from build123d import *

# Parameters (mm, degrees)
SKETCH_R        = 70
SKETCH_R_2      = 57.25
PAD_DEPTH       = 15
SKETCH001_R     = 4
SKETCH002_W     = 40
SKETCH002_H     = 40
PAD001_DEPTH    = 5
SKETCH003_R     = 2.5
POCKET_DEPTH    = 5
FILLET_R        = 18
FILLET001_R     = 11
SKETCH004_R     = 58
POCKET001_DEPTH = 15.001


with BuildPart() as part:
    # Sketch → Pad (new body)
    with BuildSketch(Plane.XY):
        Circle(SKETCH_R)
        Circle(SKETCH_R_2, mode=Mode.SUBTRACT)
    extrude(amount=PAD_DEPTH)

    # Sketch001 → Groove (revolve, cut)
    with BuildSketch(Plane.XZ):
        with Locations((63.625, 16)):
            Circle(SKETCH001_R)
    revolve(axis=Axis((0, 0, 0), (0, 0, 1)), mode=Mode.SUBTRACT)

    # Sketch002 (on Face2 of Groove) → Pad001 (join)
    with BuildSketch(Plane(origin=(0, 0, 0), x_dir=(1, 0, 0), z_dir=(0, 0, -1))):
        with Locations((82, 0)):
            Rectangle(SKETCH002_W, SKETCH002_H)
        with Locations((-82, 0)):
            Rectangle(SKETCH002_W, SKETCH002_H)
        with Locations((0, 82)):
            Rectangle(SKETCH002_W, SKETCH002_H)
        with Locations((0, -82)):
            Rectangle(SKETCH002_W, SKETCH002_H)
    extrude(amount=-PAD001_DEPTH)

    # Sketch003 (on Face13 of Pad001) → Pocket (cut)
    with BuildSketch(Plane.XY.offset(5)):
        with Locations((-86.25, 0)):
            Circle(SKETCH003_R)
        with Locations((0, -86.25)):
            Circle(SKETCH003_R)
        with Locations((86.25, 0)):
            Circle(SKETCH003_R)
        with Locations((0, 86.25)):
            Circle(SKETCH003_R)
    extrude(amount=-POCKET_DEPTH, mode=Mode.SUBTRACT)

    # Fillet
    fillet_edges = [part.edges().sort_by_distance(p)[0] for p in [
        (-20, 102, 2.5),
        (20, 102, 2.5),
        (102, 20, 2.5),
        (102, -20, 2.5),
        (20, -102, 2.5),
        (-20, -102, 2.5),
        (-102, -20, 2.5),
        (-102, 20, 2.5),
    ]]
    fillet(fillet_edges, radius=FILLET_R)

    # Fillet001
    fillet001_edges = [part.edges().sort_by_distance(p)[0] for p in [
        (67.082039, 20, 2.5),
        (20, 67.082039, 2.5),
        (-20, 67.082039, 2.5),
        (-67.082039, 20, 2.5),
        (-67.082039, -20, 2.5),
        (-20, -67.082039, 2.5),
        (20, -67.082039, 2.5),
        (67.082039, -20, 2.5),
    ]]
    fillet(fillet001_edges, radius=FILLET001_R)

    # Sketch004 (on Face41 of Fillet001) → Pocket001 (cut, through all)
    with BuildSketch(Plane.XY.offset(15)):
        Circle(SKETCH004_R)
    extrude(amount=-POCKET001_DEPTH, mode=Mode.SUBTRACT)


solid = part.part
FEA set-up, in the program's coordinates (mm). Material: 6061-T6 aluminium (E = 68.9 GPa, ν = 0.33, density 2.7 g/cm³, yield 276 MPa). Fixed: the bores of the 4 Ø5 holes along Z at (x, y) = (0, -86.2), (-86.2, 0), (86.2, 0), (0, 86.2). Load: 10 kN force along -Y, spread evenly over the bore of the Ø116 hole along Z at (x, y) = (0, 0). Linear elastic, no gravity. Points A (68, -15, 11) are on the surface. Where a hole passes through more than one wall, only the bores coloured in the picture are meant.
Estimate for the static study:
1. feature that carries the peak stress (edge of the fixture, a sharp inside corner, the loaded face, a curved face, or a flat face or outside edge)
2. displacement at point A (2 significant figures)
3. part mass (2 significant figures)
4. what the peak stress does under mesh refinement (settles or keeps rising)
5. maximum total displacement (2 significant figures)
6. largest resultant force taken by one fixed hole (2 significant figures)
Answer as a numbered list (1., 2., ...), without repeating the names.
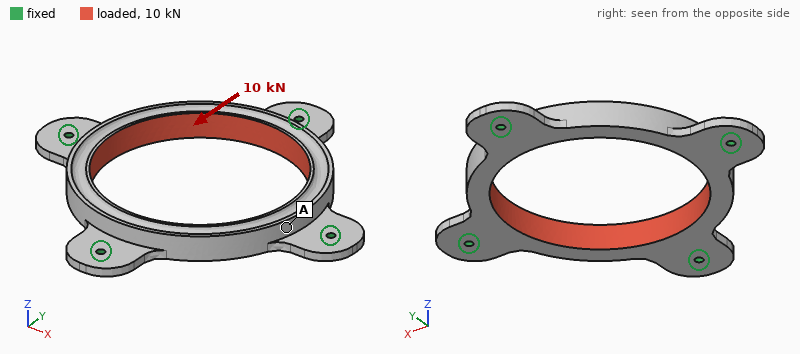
1. edge of the fixture
2. 51 µm
3. 240 g
4. keeps rising
5. 71 µm
6. 2.5 kN
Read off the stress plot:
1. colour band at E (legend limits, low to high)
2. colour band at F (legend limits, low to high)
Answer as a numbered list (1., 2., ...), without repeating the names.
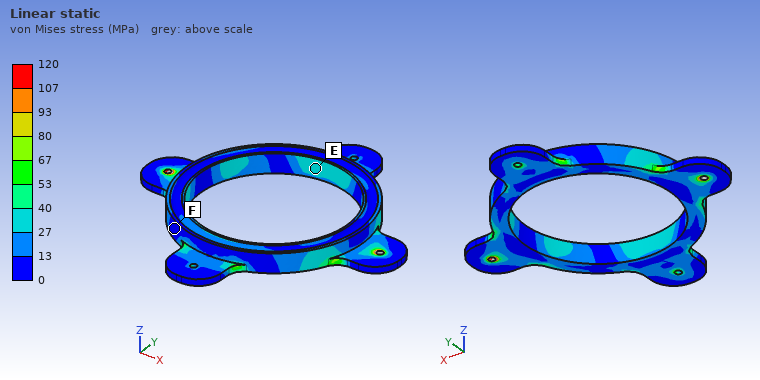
1. 27 to 40 MPa
2. 0 to 13 MPa
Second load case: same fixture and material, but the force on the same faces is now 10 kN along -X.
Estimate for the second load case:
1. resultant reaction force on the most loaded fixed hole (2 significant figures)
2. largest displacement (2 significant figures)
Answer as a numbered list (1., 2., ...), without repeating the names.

1. 2.5 kN
2. 71 µm
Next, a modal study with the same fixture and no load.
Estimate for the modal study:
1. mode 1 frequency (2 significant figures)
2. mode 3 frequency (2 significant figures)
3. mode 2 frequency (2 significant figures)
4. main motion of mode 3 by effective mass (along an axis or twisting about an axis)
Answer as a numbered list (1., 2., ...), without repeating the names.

1. 2600 Hz
2. 2900 Hz
3. 2700 Hz
4. twisting about Y
